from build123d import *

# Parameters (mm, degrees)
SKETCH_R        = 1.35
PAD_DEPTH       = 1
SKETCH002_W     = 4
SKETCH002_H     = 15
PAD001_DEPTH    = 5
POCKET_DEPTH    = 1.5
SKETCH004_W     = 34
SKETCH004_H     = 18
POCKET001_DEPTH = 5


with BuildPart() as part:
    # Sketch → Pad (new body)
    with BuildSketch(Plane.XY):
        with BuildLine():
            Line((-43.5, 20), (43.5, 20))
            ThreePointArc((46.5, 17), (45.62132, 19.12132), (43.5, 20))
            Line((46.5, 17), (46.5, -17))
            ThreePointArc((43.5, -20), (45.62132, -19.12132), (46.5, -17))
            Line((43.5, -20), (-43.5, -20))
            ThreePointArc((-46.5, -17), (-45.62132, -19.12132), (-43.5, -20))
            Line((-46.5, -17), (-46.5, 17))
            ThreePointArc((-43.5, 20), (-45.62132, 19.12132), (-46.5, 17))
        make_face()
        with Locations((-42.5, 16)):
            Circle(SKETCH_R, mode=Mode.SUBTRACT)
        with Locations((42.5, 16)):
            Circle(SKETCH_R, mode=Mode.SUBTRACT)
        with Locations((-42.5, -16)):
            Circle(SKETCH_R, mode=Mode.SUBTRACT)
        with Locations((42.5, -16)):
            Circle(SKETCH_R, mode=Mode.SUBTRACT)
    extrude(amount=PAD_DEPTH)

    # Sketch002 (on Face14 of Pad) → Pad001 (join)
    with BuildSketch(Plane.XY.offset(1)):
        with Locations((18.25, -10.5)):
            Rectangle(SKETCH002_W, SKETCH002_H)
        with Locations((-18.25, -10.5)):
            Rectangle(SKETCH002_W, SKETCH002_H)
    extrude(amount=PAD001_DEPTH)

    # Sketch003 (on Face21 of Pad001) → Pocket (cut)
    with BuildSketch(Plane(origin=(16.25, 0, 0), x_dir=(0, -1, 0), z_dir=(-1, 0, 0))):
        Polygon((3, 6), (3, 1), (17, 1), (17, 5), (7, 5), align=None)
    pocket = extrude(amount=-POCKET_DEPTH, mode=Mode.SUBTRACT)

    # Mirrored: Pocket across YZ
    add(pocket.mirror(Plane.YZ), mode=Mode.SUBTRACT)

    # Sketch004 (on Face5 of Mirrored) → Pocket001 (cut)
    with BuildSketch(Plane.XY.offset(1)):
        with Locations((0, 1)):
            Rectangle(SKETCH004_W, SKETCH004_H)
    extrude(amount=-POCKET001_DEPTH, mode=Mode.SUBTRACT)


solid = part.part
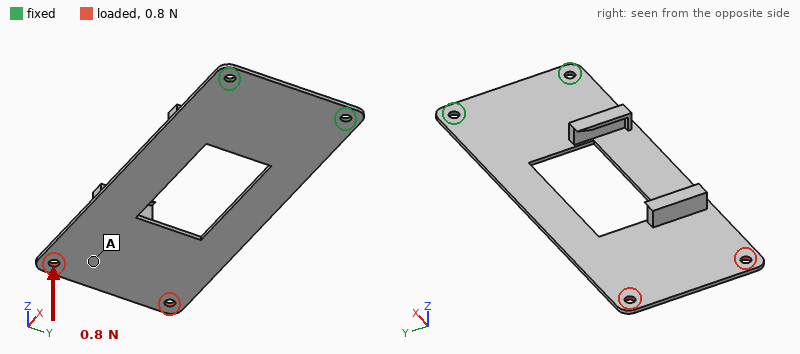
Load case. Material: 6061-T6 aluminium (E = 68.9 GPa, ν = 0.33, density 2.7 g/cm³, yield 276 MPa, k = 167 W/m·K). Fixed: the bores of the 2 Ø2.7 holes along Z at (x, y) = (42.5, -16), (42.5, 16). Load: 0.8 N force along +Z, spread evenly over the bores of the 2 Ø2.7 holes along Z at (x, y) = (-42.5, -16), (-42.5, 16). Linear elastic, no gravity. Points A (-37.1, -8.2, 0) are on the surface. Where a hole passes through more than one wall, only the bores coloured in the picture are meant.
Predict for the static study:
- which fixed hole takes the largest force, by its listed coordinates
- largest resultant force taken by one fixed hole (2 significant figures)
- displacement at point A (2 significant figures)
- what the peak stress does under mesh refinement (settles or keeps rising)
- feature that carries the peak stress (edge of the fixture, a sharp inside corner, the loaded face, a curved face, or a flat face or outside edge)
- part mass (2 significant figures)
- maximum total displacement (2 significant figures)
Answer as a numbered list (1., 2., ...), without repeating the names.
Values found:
1. (42.5, 16)
2. 0.45 N
3. 0.84 mm
4. keeps rising
5. edge of the fixture
6. 9.5 g
7. 1.0 mm
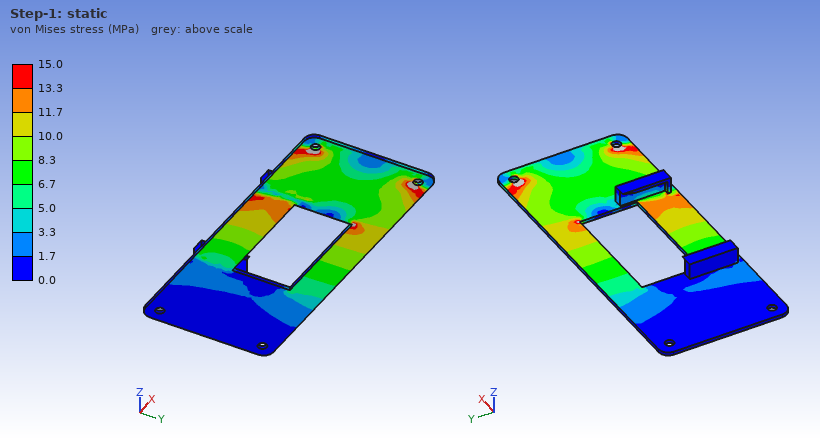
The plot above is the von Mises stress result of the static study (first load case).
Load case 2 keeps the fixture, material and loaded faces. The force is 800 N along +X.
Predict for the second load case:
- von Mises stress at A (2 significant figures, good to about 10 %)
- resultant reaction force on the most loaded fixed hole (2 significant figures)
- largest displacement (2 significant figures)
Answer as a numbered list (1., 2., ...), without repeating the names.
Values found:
1. 13 MPa
2. 410 N
3. 67 µm
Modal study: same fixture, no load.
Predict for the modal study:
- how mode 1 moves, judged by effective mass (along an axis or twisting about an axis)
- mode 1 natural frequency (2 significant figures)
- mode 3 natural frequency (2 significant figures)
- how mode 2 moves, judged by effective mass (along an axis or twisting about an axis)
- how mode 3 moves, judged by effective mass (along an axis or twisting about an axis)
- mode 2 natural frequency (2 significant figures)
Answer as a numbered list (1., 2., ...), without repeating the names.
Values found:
1. along Z
2. 92 Hz
3. 600 Hz
4. twisting about X
5. along Z
6. 440 Hz
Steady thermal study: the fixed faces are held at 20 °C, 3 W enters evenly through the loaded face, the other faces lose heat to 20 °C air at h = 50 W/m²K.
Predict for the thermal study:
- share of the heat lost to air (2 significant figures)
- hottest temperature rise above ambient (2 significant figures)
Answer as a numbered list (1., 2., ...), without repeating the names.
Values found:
1. 85 %
2. 22 K
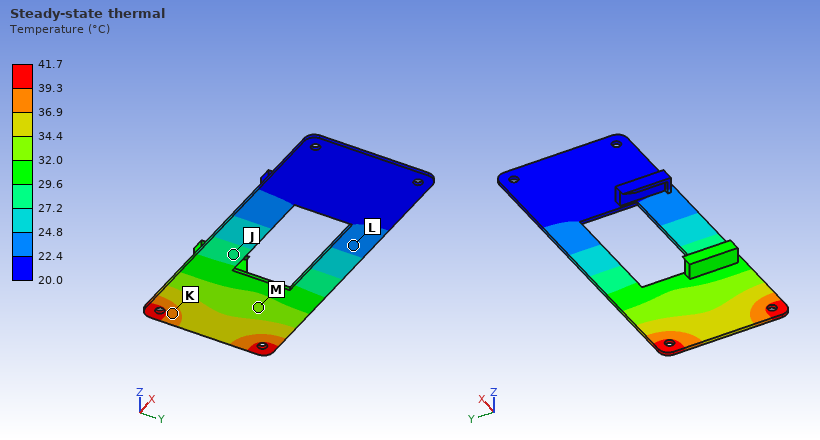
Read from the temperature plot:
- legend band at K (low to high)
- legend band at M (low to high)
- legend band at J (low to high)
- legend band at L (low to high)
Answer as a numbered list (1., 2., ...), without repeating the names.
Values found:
1. 36.9 to 39.3 °C
2. 32.0 to 34.4 °C
3. 27.2 to 29.6 °C
4. 22.4 to 24.8 °C
